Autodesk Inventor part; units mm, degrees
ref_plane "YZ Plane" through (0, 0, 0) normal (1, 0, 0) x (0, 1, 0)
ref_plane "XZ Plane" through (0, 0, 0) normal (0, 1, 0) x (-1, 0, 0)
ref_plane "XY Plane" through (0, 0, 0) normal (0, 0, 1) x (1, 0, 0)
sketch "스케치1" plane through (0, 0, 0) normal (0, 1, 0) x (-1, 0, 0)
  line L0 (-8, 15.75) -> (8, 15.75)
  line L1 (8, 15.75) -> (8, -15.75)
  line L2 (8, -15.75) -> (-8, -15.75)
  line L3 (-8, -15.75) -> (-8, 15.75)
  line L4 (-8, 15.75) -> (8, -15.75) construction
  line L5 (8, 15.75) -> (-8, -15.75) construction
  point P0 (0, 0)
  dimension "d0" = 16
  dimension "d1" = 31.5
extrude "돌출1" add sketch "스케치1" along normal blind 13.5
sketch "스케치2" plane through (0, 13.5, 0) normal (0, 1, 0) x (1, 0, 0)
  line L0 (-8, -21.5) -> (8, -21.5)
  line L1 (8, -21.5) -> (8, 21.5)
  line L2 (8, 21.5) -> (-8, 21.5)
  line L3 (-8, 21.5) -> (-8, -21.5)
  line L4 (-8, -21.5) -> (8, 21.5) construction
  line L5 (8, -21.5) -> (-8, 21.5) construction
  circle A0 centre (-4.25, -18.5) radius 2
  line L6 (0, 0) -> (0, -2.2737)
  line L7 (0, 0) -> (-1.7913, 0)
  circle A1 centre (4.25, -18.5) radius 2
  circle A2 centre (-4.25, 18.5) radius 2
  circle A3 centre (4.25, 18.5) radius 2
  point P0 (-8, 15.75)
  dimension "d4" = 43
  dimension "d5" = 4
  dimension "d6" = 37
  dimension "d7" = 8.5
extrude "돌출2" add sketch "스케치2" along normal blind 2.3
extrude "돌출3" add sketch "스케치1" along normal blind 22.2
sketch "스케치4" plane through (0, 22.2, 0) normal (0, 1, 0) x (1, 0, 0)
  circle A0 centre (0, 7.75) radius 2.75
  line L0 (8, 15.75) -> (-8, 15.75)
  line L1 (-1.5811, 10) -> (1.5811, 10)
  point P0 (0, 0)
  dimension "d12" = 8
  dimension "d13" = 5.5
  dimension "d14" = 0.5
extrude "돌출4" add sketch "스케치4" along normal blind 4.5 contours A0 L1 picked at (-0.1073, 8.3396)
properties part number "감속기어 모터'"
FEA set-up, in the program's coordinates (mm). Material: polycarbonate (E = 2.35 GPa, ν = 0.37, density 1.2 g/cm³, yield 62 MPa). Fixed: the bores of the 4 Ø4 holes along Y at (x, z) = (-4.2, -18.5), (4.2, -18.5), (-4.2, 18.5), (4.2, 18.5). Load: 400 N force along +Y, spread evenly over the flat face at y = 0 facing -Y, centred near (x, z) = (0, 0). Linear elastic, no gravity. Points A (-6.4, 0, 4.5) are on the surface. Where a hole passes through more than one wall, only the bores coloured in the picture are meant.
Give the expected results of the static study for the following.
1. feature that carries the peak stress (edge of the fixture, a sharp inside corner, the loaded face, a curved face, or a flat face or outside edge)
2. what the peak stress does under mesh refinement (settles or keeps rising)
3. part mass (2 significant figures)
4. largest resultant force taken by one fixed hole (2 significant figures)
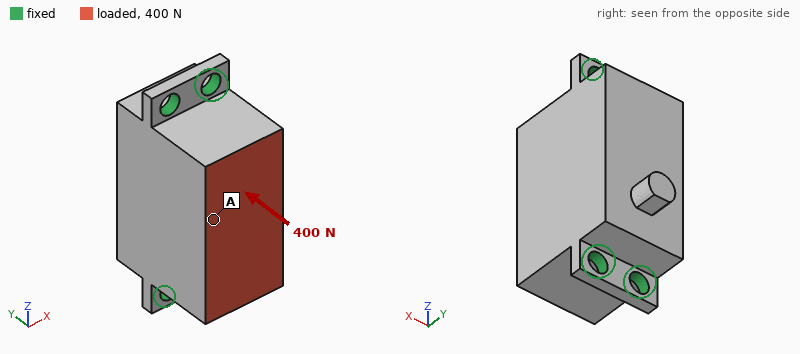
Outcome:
edge of the fixture
keeps rising
14 g
100 N
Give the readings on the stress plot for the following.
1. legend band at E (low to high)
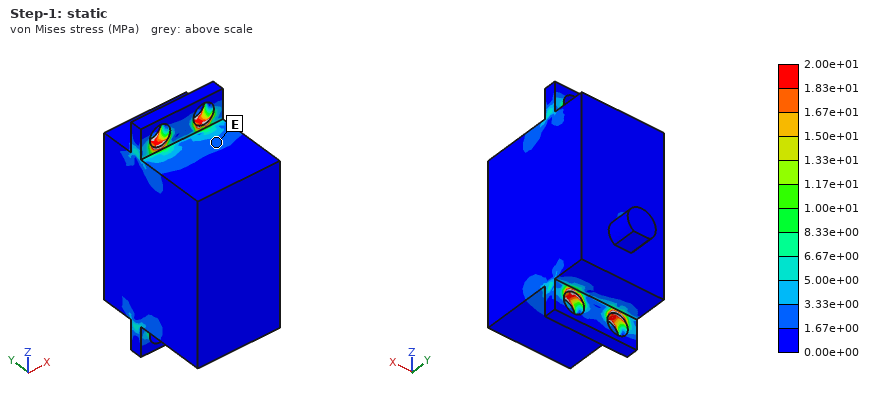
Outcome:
1.67e+00 to 3.33e+00 MPa
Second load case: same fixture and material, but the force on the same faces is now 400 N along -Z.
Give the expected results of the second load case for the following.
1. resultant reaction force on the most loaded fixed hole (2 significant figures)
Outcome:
140 N
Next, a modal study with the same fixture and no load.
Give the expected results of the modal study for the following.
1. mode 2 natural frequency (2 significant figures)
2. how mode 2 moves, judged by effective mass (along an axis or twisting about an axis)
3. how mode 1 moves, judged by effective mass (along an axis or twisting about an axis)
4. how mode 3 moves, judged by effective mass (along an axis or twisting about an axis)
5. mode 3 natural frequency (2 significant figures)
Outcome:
5200 Hz
along Y
along X
along X
5700 Hz
